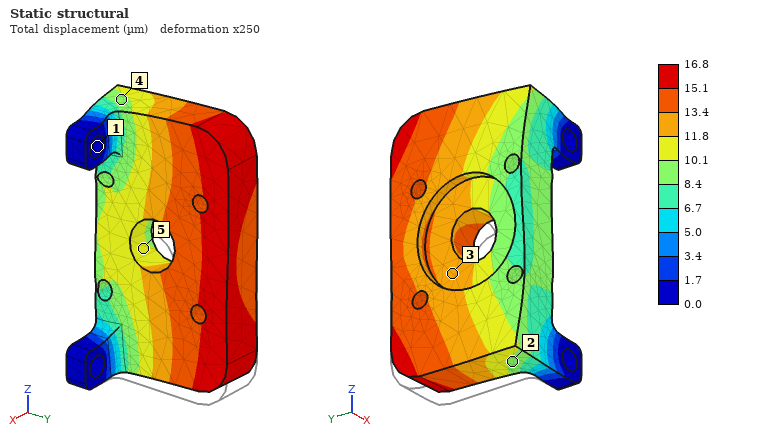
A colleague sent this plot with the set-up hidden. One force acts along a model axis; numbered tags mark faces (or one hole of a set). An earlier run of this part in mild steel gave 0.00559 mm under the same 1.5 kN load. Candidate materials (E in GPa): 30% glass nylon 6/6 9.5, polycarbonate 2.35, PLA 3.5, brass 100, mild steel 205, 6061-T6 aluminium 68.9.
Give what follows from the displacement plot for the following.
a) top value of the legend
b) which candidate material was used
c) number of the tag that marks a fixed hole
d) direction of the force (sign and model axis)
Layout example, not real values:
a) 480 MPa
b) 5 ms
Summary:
a) 16.8 µm
b) 6061-T6 aluminium
c) 1
d) +Z
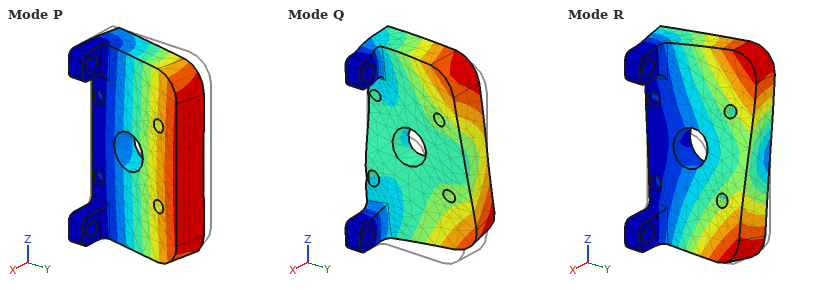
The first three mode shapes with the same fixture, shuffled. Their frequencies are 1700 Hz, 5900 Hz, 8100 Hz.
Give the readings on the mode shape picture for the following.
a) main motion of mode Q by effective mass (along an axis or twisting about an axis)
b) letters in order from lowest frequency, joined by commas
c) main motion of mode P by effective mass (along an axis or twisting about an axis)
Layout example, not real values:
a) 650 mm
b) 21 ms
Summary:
a) along Z
b) P, R, Q
c) along X
